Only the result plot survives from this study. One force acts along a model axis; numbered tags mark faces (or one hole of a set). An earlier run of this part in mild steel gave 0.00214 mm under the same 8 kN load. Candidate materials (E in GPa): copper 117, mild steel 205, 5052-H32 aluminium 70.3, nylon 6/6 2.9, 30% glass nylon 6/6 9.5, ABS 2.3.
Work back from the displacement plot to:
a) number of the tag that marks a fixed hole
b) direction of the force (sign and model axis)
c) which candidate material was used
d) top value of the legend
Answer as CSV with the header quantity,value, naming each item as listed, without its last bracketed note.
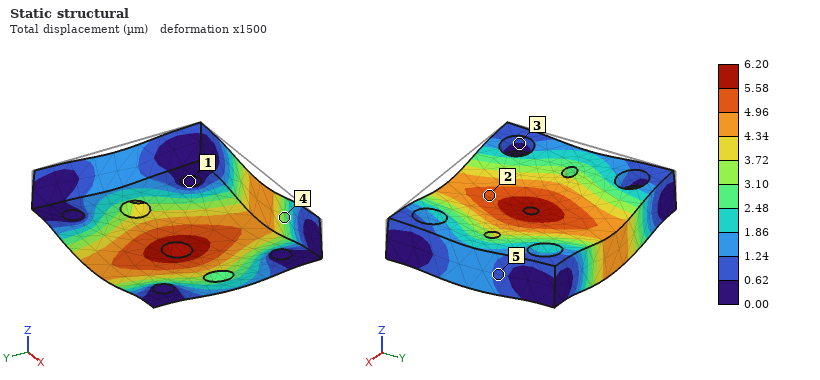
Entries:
quantity,value
number of the tag that marks a fixed hole,1
direction of the force,-Z
which candidate material was used,5052-H32 aluminium
top value of the legend,6.20 µm
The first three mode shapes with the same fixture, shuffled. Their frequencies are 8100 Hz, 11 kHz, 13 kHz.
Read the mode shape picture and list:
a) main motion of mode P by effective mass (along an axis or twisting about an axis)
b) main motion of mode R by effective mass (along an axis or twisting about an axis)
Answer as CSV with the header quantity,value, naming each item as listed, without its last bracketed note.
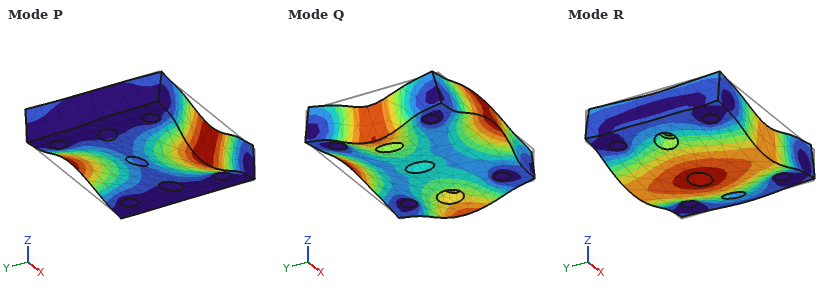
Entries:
quantity,value
main motion of mode P by effective mass,twisting about X
main motion of mode R by effective mass,along Z
